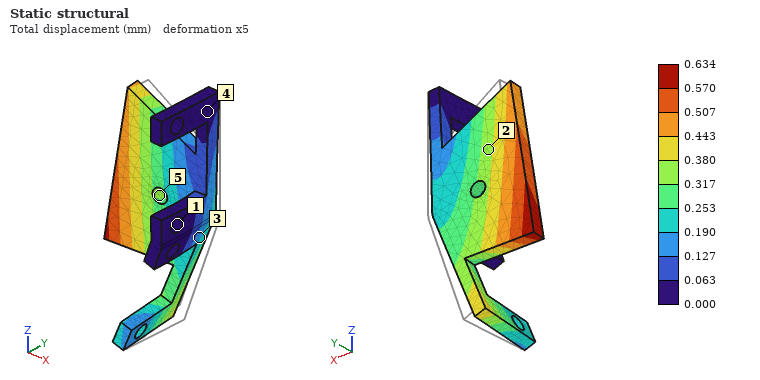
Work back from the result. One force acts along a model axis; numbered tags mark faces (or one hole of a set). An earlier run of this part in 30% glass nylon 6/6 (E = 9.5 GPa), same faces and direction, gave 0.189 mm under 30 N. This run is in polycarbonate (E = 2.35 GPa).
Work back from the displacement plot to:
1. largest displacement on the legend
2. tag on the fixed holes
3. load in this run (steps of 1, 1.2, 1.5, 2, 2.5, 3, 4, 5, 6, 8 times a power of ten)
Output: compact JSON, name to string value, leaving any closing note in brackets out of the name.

{"largest displacement on the legend": "0.634 mm", "tag on the fixed holes": "1", "load in this run": "25 N"}
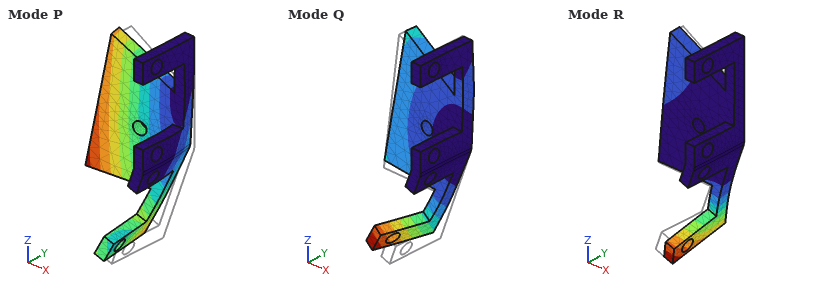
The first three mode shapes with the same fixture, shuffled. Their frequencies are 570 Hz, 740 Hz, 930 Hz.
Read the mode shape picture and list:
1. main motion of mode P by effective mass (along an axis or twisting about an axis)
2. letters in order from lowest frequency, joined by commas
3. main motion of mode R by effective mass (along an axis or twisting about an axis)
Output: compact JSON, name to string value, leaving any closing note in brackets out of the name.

{"main motion of mode P by effective mass": "along Y", "letters in order from lowest frequency, joined by commas": "P, Q, R", "main motion of mode R by effective mass": "twisting about X"}
